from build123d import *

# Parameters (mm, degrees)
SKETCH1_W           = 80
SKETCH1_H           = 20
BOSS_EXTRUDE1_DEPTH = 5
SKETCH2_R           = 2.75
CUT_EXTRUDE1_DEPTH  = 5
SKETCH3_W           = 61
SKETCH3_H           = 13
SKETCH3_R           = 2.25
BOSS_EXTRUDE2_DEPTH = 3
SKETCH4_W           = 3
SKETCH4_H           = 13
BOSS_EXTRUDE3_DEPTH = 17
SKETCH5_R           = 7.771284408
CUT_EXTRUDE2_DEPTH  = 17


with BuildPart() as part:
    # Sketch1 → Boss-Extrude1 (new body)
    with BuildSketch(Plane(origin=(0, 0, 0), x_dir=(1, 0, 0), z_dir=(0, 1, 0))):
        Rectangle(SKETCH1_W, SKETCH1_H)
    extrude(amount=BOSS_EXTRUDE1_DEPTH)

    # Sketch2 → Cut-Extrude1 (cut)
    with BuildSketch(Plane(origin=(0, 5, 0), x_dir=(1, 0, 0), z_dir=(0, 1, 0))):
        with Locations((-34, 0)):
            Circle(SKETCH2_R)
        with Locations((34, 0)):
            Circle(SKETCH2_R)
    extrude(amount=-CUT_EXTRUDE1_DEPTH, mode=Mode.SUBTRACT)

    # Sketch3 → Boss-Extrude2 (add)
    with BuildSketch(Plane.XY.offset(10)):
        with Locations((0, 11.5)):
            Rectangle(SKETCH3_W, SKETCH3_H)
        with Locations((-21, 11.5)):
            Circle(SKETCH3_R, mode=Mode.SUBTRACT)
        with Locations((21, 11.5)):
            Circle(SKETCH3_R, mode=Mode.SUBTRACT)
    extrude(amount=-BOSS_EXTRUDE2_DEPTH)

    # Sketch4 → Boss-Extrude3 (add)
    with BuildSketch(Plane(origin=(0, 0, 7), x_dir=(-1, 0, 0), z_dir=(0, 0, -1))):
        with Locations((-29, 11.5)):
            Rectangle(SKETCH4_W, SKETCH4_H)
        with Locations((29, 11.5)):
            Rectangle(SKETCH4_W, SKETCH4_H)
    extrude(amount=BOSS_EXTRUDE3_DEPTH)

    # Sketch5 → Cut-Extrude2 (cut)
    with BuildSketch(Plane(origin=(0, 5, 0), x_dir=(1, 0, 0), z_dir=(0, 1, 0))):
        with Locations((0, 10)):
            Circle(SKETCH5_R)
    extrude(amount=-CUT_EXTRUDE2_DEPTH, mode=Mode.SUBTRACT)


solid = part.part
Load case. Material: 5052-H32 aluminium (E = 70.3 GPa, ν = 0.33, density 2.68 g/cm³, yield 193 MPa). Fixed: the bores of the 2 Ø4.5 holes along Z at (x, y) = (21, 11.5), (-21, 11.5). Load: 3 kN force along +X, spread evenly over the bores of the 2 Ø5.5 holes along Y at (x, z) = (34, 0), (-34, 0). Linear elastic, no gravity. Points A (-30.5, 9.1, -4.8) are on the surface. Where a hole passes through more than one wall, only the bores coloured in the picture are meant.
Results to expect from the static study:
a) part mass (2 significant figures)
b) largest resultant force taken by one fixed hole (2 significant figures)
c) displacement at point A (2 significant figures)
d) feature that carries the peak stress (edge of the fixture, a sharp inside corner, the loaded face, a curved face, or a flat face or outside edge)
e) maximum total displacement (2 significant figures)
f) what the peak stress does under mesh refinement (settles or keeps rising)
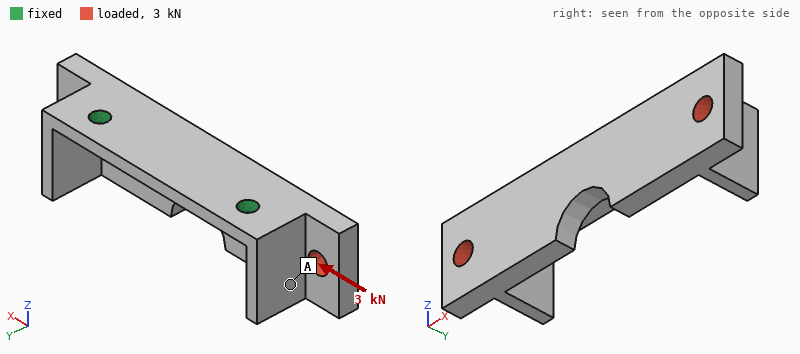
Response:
29 g
1.7 kN
34 µm
edge of the fixture
61 µm
keeps rising
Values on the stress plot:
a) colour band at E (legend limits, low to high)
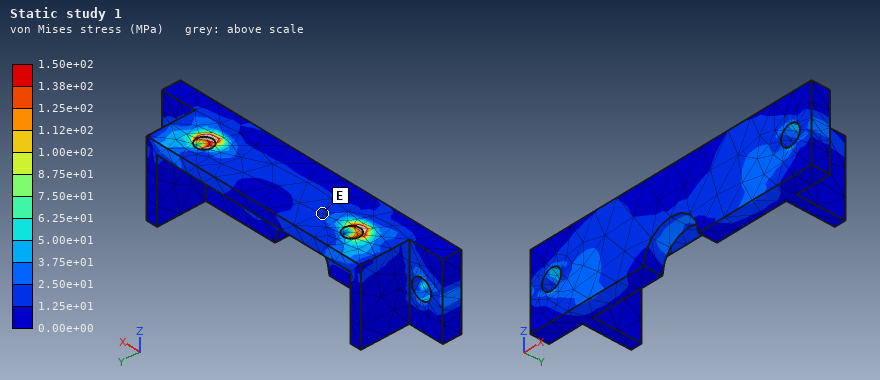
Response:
1.25e+01 to 2.50e+01 MPa
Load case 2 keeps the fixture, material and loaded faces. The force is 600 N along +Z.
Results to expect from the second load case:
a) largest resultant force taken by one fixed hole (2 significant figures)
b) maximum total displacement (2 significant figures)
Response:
330 N
50 µm
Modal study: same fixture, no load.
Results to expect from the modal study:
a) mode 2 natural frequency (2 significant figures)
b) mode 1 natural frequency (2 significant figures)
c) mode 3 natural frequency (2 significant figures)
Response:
5000 Hz
4000 Hz
8600 Hz
